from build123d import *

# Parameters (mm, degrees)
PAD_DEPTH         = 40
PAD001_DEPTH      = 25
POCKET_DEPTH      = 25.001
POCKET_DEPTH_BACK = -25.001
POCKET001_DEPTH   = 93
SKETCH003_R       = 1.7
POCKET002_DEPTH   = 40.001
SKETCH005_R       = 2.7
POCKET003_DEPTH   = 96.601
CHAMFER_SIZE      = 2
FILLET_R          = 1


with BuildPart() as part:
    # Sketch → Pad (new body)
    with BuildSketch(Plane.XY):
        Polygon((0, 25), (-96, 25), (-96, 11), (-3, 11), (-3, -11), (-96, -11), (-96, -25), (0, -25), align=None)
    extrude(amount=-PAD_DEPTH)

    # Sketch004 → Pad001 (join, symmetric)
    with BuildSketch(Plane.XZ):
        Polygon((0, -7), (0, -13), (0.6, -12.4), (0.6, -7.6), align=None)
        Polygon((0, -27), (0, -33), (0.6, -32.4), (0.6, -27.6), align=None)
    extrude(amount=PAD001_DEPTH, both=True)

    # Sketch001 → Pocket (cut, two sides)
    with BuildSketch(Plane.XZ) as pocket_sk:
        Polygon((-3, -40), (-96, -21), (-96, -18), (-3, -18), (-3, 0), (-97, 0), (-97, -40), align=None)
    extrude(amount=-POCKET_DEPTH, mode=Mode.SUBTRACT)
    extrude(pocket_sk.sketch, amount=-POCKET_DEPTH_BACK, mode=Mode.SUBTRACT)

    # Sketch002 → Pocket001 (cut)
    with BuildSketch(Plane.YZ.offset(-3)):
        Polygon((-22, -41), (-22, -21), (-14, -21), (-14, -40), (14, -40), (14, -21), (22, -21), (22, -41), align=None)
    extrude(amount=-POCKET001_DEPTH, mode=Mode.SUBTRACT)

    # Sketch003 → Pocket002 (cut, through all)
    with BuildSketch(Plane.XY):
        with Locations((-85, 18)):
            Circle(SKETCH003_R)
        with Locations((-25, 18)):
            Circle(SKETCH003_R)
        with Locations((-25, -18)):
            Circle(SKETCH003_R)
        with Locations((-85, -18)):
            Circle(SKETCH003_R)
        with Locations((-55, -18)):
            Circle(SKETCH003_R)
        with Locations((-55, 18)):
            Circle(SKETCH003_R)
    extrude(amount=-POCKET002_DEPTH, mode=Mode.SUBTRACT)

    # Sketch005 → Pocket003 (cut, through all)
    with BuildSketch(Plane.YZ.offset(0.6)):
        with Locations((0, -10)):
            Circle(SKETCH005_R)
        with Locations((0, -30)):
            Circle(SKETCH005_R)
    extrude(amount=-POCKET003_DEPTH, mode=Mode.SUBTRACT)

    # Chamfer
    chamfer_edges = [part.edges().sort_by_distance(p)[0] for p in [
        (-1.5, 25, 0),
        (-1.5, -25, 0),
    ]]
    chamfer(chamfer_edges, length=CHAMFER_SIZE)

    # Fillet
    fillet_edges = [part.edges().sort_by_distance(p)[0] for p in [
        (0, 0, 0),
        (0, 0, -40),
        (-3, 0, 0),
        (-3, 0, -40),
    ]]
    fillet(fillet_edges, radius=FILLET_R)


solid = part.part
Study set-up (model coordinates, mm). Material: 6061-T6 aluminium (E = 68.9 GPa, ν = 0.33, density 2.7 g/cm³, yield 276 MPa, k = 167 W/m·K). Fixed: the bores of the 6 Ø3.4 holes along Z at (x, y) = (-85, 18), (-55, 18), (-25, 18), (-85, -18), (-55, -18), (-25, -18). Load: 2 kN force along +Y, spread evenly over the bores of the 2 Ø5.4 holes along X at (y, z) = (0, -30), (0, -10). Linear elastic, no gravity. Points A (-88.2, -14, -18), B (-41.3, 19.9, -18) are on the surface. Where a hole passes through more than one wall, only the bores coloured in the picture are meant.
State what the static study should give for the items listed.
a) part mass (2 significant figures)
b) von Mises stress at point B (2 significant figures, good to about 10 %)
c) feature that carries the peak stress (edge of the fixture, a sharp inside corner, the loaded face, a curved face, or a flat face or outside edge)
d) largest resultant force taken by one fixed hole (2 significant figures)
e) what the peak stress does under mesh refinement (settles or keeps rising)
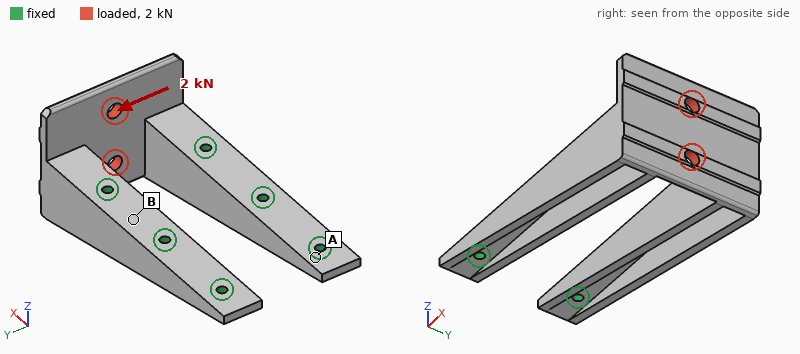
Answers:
66 g
17 MPa
edge of the fixture
1.4 kN
keeps rising
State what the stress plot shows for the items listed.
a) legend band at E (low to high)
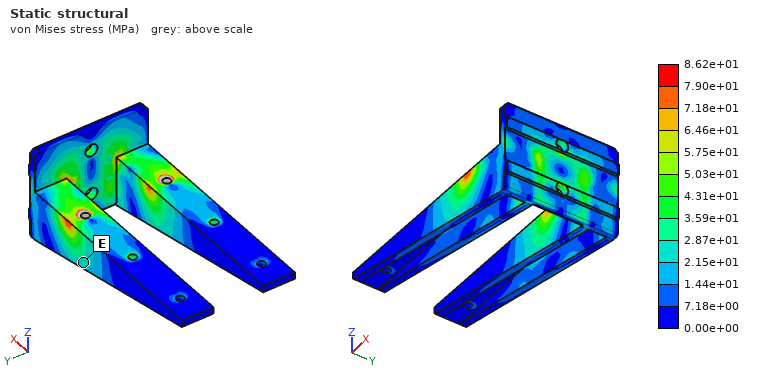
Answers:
2.15e+01 to 2.87e+01 MPa
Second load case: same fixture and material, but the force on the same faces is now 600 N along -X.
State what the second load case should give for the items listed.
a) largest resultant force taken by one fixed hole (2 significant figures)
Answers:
270 N
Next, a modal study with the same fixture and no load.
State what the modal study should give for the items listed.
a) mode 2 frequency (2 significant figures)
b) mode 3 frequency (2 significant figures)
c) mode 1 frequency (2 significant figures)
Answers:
5000 Hz
5800 Hz
4800 Hz
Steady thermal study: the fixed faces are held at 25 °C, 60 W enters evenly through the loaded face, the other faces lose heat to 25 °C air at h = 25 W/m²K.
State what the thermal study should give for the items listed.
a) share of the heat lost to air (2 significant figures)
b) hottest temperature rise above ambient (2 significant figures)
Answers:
13 %
69 K
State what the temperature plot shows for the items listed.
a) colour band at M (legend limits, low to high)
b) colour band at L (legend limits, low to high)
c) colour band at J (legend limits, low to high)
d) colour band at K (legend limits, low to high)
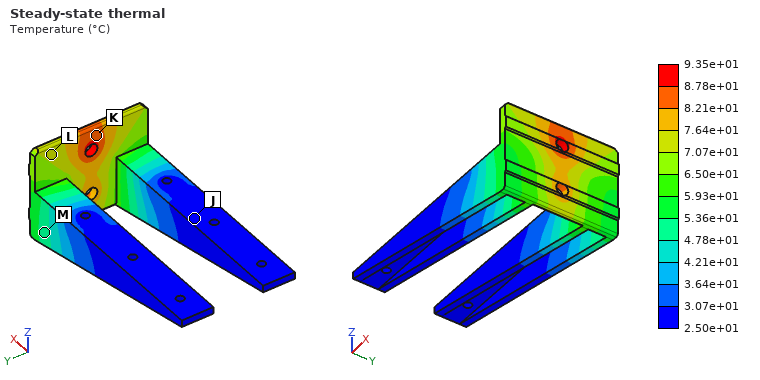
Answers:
4.78e+01 to 5.36e+01 °C
7.07e+01 to 7.64e+01 °C
2.50e+01 to 3.07e+01 °C
8.21e+01 to 8.78e+01 °C
